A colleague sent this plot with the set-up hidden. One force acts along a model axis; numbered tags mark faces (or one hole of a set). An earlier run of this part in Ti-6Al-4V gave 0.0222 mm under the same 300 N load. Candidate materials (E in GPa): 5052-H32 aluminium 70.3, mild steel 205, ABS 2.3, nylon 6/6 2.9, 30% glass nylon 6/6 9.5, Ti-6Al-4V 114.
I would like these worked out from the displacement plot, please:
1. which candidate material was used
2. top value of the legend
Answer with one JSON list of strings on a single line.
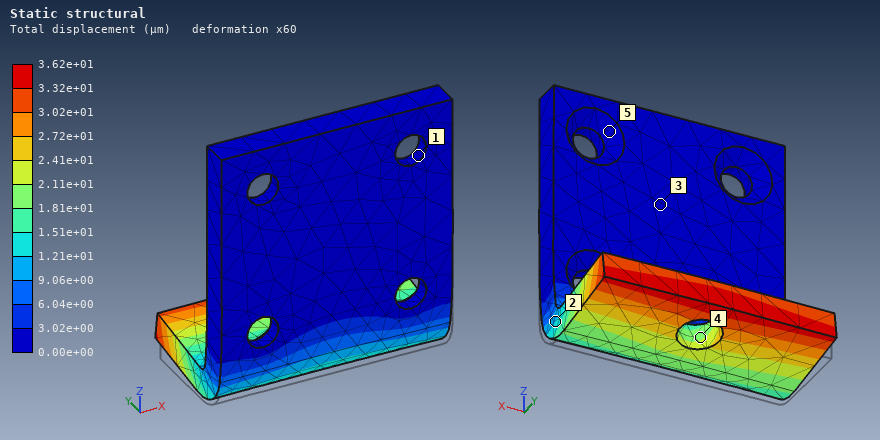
["5052-H32 aluminium", "3.62e+01 µm"]
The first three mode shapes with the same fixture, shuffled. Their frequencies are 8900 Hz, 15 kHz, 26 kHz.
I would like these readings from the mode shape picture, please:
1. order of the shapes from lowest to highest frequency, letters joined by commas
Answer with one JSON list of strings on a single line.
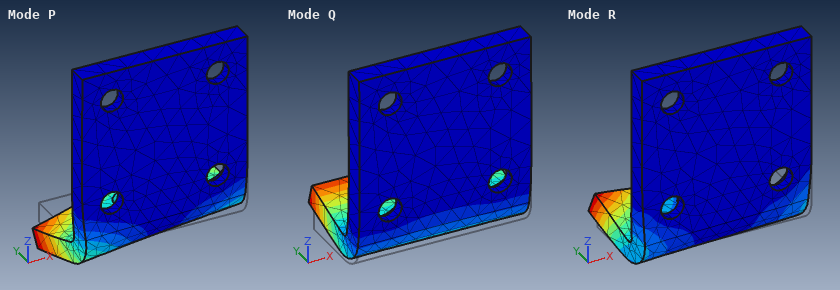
["Q, P, R"]
